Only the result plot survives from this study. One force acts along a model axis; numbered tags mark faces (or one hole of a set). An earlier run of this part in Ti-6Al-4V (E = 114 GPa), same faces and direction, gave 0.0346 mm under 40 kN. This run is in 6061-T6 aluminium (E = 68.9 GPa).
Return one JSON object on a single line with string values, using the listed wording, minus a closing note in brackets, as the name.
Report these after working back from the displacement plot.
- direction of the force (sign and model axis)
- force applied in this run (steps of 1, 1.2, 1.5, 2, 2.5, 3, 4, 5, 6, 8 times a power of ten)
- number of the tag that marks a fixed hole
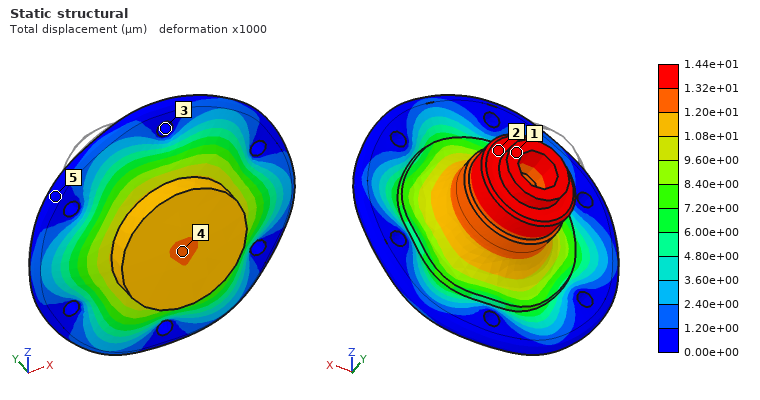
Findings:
{"direction of the force": "-Y", "force applied in this run": "10 kN", "number of the tag that marks a fixed hole": "3"}
